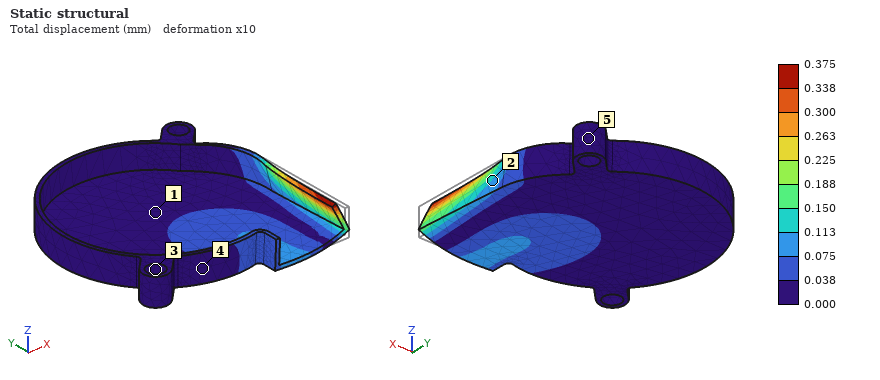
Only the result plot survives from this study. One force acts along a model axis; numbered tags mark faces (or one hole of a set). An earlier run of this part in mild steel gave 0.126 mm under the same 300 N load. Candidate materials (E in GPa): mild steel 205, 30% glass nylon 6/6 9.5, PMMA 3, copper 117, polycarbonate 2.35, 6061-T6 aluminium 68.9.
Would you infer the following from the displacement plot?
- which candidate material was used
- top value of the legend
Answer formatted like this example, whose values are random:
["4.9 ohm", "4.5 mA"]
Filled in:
["6061-T6 aluminium", "0.375 mm"]
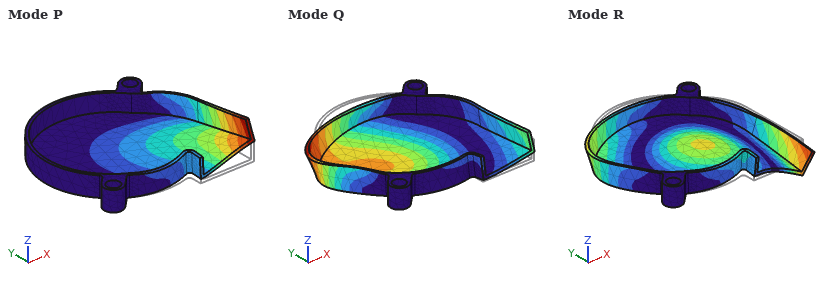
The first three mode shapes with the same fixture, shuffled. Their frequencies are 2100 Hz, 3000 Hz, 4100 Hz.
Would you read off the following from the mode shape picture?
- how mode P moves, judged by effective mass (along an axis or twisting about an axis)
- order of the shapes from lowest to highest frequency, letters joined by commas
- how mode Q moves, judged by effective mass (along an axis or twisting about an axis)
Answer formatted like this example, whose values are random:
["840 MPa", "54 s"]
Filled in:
["along Z", "P, Q, R", "along Z"]
